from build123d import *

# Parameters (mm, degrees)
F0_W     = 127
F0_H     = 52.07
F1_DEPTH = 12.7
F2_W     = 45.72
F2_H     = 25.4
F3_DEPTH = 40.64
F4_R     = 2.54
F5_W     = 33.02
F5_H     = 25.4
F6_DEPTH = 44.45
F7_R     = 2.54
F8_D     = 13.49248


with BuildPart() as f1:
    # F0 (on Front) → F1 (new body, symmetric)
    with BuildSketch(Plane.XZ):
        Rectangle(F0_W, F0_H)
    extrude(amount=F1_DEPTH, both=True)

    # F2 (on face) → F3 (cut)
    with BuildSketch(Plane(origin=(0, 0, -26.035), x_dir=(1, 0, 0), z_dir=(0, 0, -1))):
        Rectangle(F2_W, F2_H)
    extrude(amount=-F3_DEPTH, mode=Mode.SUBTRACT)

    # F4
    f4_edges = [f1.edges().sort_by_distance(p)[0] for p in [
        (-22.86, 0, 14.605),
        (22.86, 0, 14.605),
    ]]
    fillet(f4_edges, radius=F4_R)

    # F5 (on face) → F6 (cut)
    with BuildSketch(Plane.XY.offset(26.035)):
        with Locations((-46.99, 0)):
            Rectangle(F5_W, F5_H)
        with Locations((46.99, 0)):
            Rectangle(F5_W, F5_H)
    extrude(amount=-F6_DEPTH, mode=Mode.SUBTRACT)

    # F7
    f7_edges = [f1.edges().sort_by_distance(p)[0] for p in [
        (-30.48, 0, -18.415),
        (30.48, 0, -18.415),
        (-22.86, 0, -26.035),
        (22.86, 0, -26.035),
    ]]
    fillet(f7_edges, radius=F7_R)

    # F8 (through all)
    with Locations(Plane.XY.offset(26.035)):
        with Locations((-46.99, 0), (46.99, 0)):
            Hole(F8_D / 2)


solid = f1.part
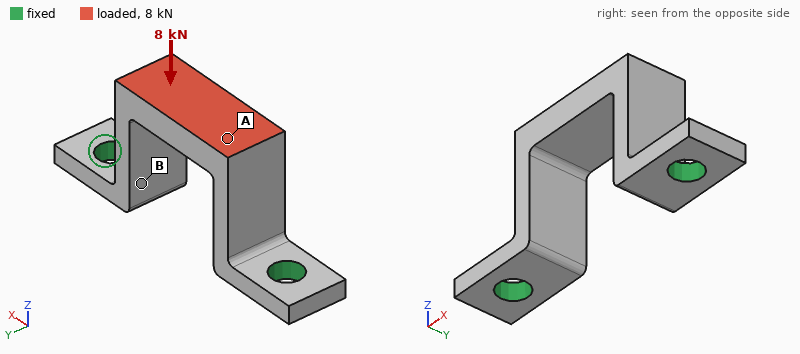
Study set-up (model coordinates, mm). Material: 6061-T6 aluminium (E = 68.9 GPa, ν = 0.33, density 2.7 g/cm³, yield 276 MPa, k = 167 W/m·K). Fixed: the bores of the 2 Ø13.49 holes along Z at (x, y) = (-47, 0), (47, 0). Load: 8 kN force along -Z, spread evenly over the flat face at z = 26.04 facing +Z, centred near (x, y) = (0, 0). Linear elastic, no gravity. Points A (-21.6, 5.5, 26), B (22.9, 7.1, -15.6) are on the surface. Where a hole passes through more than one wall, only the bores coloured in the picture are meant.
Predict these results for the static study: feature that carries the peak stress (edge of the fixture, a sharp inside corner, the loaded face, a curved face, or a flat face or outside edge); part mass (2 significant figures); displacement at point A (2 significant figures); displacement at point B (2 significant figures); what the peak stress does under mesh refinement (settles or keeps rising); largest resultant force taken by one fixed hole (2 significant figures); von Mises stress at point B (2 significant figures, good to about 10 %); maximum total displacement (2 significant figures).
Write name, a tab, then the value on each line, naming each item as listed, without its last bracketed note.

feature that carries the peak stress	edge of the fixture
part mass	120 g
displacement at point A	59 µm
displacement at point B	47 µm
what the peak stress does under mesh refinement	keeps rising
largest resultant force taken by one fixed hole	4.2 kN
von Mises stress at point B	43 MPa
maximum total displacement	81 µm
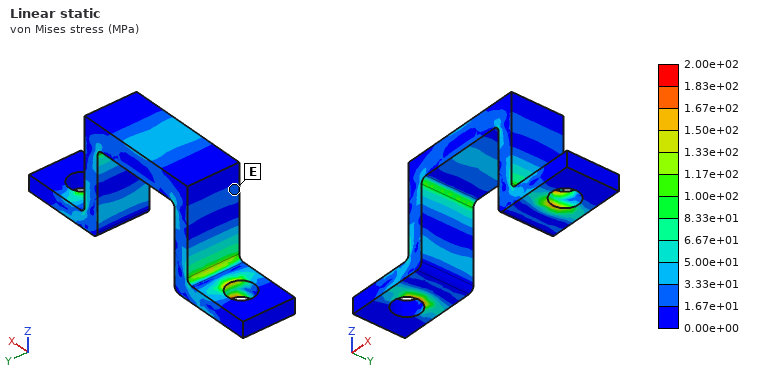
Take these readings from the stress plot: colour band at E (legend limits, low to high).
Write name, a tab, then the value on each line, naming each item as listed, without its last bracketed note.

colour band at E	1.67e+01 to 3.33e+01 MPa
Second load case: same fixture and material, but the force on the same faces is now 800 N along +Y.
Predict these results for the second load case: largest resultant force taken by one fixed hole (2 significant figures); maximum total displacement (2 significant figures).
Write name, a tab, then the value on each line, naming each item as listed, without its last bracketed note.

largest resultant force taken by one fixed hole	400 N
maximum total displacement	0.13 mm
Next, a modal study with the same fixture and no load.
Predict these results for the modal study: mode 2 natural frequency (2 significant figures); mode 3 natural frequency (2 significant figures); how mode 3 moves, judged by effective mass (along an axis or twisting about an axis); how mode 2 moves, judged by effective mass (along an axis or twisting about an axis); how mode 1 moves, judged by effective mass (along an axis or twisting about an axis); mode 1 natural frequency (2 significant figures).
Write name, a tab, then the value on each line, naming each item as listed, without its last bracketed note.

mode 2 natural frequency	2700 Hz
mode 3 natural frequency	4000 Hz
how mode 3 moves, judged by effective mass	twisting about Z
how mode 2 moves, judged by effective mass	along X
how mode 1 moves, judged by effective mass	along Y
mode 1 natural frequency	1800 Hz
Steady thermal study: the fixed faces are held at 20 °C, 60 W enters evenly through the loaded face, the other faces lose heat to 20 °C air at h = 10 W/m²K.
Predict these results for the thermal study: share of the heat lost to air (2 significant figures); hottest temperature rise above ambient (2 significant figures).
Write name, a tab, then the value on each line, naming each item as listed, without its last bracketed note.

share of the heat lost to air	4.9 %
hottest temperature rise above ambient	53 K
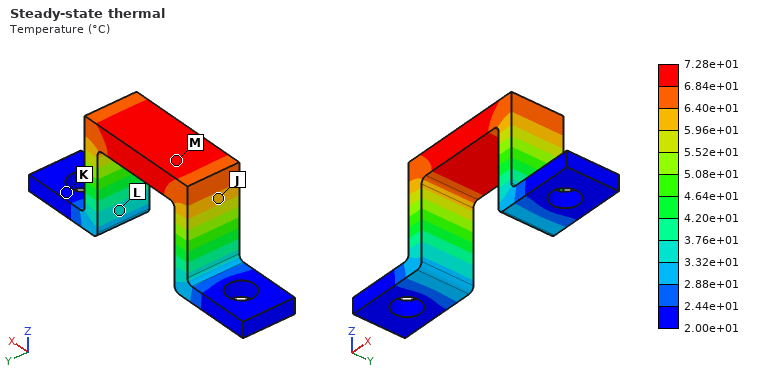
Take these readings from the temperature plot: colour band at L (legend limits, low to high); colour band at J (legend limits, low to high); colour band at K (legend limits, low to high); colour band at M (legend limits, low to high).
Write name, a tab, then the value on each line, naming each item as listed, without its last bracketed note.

colour band at L	3.32e+01 to 3.76e+01 °C
colour band at J	5.96e+01 to 6.40e+01 °C
colour band at K	2.00e+01 to 2.44e+01 °C
colour band at M	6.84e+01 to 7.28e+01 °C
